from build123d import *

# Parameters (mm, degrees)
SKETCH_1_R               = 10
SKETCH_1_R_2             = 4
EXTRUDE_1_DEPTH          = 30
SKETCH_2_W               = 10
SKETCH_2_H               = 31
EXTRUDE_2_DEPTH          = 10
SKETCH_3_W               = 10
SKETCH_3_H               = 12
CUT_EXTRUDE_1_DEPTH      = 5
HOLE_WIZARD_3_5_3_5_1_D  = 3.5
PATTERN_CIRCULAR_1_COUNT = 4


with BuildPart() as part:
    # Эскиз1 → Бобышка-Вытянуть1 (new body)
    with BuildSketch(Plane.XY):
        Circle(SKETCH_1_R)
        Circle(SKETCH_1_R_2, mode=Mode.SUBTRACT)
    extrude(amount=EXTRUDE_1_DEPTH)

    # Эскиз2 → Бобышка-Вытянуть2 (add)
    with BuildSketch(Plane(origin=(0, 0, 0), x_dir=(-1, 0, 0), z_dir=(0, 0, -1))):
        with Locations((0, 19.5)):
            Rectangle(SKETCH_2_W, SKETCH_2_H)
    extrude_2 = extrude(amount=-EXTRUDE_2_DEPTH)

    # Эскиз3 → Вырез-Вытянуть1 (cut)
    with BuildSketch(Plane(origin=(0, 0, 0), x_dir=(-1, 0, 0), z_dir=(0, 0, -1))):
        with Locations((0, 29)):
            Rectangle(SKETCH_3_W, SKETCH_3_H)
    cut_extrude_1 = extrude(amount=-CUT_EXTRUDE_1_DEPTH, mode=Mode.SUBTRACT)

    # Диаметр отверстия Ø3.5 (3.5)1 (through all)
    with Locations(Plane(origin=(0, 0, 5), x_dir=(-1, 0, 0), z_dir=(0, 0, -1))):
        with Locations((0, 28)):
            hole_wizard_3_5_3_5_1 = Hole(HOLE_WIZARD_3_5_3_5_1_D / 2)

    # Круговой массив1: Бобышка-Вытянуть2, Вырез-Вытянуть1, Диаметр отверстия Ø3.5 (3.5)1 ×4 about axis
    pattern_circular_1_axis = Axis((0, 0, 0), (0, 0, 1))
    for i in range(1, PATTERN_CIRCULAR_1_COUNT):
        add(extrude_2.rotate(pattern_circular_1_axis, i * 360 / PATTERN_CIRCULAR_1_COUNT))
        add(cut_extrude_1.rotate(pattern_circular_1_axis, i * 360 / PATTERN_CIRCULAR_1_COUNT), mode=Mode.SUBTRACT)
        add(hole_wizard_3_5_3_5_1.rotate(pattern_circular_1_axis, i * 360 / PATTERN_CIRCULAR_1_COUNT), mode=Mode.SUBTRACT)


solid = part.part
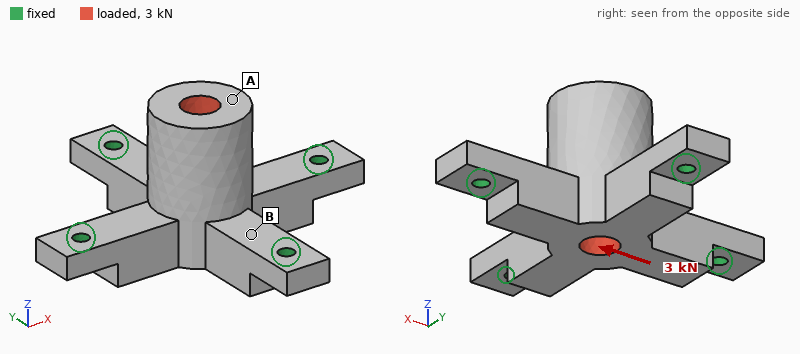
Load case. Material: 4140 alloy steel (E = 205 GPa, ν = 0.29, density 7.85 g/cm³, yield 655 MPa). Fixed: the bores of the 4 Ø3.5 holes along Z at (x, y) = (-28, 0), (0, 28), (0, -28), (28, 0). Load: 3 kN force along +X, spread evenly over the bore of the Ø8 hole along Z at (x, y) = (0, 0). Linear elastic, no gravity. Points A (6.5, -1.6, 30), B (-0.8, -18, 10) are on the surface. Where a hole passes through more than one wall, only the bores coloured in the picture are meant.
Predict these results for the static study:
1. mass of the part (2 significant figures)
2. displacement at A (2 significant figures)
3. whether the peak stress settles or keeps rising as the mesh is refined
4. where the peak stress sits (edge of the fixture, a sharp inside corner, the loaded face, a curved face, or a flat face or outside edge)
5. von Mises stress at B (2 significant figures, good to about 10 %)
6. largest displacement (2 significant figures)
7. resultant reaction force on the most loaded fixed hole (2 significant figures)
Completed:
120 g
15 µm
keeps rising
edge of the fixture
20 MPa
16 µm
1.4 kN
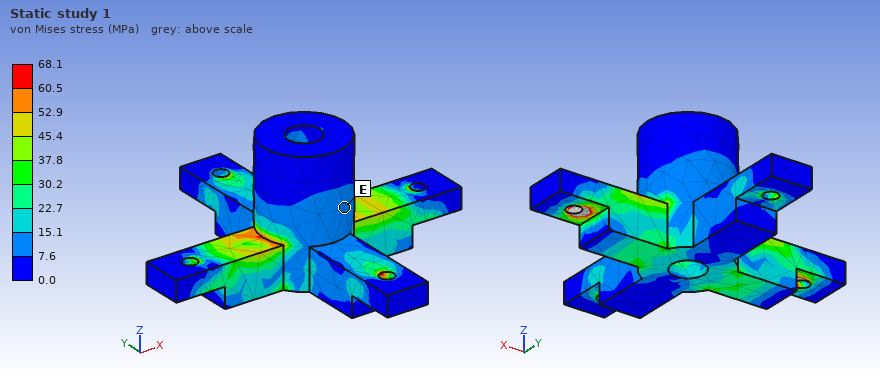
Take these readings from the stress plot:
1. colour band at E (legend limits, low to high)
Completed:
7.6 to 15.1 MPa
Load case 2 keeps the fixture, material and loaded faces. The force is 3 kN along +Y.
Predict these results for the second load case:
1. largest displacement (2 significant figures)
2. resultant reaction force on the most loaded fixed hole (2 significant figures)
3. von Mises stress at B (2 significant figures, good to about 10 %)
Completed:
16 µm
1.4 kN
46 MPa
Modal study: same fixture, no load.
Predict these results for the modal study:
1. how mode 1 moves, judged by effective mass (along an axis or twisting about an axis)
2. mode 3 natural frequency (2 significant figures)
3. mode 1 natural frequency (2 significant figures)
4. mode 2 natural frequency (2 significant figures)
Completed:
along Z
10 kHz
9700 Hz
10 kHz
